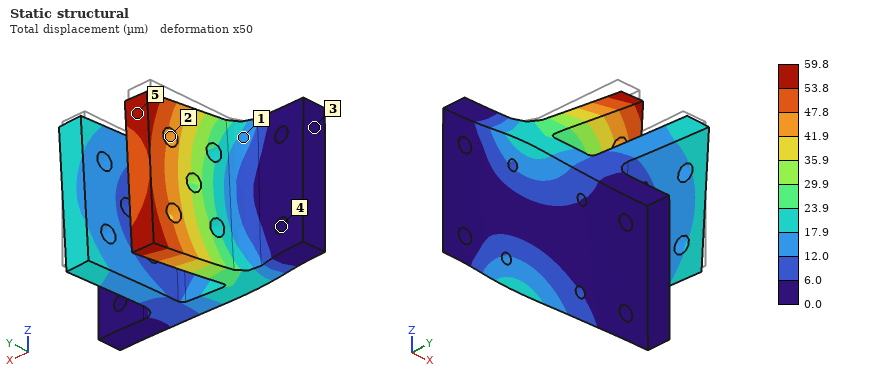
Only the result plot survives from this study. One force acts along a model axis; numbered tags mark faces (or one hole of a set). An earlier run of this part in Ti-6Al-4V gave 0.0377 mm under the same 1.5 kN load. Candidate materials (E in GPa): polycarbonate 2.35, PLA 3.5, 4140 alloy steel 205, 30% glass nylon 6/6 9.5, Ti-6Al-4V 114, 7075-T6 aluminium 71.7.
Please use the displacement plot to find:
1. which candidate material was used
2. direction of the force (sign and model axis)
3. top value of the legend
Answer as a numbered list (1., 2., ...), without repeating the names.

1. 7075-T6 aluminium
2. -Z
3. 59.8 µm
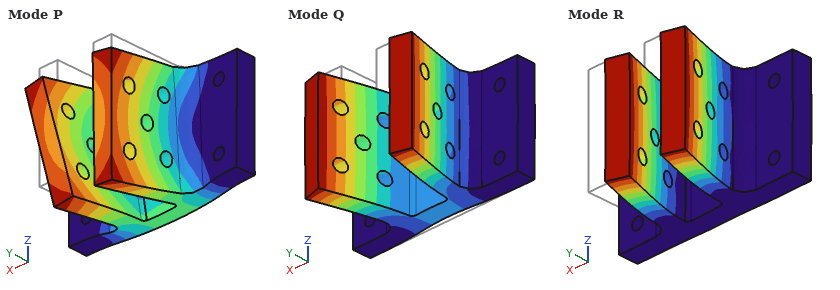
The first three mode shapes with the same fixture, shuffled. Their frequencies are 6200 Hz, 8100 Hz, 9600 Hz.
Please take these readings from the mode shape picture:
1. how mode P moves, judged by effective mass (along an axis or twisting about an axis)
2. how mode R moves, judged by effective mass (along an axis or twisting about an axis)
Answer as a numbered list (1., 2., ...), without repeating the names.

1. along Z
2. along X
